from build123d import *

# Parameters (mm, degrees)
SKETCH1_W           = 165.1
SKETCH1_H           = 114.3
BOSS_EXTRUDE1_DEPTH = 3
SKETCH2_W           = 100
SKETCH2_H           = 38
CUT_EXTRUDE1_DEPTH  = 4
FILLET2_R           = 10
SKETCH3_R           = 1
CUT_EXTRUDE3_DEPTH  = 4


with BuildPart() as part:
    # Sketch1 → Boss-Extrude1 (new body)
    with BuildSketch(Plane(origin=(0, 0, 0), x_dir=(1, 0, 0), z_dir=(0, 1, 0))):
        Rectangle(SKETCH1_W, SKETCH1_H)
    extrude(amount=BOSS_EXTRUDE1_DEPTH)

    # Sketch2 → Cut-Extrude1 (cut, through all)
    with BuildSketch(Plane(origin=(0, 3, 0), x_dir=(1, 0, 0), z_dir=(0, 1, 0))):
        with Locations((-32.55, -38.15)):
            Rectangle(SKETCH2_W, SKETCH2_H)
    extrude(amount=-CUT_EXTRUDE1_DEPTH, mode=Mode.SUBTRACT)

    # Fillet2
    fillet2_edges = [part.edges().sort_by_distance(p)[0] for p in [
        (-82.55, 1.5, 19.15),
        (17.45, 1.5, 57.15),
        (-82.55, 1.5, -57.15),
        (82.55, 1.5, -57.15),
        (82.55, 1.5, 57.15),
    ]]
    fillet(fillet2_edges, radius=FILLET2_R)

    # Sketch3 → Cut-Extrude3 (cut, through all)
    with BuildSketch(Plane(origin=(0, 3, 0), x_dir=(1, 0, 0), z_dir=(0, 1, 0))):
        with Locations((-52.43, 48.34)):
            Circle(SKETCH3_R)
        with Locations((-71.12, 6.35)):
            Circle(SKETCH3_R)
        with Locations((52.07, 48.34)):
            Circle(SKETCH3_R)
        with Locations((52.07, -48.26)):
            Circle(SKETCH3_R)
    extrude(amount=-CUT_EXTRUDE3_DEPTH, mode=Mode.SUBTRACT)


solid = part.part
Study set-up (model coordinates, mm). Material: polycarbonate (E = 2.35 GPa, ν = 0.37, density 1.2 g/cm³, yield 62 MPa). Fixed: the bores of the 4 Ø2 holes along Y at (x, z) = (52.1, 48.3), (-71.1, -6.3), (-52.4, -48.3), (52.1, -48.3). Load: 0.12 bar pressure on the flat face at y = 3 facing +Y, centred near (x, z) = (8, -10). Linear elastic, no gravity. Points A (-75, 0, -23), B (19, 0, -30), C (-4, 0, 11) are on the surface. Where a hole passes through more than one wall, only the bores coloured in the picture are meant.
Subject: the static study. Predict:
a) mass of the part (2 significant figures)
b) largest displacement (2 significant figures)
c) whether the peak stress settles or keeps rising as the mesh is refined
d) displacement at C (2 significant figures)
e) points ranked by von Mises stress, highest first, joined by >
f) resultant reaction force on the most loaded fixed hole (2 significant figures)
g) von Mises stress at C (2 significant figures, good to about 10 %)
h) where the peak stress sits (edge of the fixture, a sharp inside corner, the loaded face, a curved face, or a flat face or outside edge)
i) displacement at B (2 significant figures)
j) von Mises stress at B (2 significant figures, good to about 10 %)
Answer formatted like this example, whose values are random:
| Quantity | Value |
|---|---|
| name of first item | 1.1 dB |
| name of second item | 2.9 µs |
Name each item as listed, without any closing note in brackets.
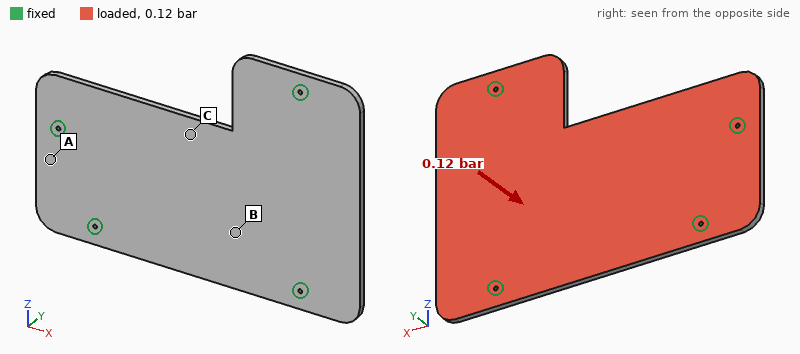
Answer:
| Quantity | Value |
|---|---|
| mass of the part | 54 g |
| largest displacement | 2.3 mm |
| whether the peak stress settles or keeps rising as the mesh is refined | keeps rising |
| displacement at C | 2.2 mm |
| points ranked by von Mises stress, highest first, joined by > | C > B > A |
| resultant reaction force on the most loaded fixed hole | 56 N |
| von Mises stress at C | 5.6 MPa |
| where the peak stress sits | edge of the fixture |
| displacement at B | 1.3 mm |
| von Mises stress at B | 3.1 MPa |
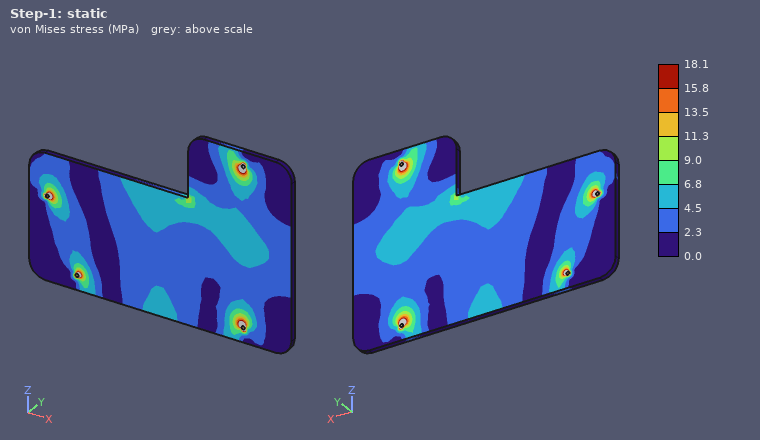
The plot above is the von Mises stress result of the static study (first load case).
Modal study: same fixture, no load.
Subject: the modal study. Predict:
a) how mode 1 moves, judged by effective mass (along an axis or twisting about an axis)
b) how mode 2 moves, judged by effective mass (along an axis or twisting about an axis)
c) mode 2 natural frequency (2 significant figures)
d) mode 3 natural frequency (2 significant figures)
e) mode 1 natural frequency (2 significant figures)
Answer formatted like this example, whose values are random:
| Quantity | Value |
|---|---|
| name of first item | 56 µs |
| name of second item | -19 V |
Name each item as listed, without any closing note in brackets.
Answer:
| Quantity | Value |
|---|---|
| how mode 1 moves, judged by effective mass | along Y |
| how mode 2 moves, judged by effective mass | along Y |
| mode 2 natural frequency | 330 Hz |
| mode 3 natural frequency | 440 Hz |
| mode 1 natural frequency | 240 Hz |
